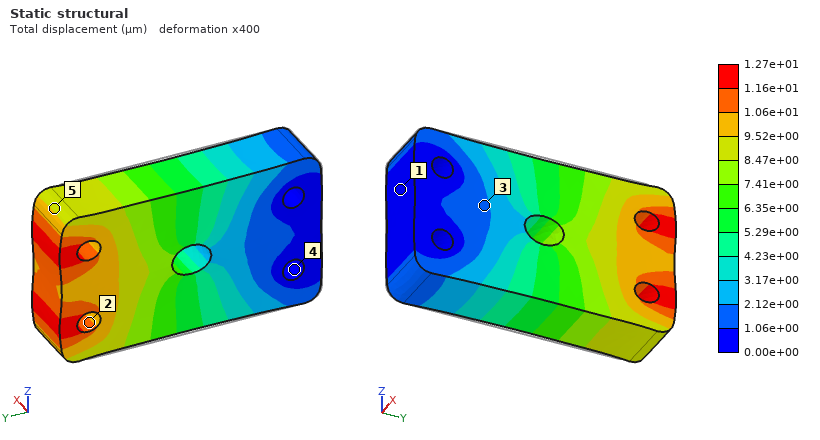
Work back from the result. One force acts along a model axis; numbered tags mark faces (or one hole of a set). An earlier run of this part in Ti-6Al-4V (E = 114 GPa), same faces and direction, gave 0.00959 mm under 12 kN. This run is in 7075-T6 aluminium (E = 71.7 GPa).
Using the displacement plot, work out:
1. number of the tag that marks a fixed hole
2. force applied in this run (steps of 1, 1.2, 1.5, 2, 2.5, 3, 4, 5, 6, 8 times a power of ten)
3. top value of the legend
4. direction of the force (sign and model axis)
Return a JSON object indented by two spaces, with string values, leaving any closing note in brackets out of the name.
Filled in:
{
  "number of the tag that marks a fixed hole": "4",
  "force applied in this run": "10 kN",
  "top value of the legend": "1.27e+01 µm",
  "direction of the force": "+Y"
}
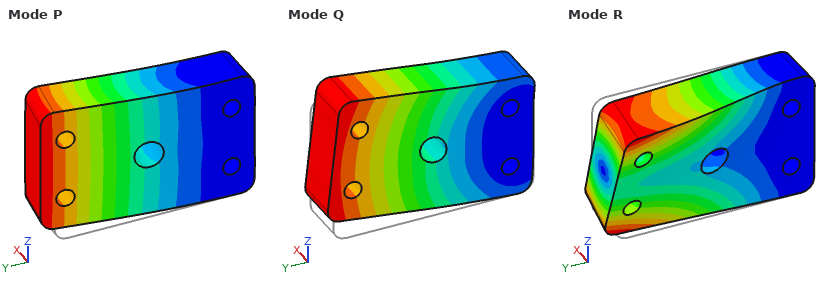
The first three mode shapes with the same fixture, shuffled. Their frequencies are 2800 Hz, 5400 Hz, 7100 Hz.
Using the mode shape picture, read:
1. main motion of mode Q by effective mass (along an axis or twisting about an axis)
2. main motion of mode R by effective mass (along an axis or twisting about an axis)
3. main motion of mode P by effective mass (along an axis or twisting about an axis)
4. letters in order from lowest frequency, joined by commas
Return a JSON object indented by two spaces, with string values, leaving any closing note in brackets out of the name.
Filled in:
{
  "main motion of mode Q by effective mass": "along Z",
  "main motion of mode R by effective mass": "twisting about Y",
  "main motion of mode P by effective mass": "along X",
  "letters in order from lowest frequency, joined by commas": "P, Q, R"
}
